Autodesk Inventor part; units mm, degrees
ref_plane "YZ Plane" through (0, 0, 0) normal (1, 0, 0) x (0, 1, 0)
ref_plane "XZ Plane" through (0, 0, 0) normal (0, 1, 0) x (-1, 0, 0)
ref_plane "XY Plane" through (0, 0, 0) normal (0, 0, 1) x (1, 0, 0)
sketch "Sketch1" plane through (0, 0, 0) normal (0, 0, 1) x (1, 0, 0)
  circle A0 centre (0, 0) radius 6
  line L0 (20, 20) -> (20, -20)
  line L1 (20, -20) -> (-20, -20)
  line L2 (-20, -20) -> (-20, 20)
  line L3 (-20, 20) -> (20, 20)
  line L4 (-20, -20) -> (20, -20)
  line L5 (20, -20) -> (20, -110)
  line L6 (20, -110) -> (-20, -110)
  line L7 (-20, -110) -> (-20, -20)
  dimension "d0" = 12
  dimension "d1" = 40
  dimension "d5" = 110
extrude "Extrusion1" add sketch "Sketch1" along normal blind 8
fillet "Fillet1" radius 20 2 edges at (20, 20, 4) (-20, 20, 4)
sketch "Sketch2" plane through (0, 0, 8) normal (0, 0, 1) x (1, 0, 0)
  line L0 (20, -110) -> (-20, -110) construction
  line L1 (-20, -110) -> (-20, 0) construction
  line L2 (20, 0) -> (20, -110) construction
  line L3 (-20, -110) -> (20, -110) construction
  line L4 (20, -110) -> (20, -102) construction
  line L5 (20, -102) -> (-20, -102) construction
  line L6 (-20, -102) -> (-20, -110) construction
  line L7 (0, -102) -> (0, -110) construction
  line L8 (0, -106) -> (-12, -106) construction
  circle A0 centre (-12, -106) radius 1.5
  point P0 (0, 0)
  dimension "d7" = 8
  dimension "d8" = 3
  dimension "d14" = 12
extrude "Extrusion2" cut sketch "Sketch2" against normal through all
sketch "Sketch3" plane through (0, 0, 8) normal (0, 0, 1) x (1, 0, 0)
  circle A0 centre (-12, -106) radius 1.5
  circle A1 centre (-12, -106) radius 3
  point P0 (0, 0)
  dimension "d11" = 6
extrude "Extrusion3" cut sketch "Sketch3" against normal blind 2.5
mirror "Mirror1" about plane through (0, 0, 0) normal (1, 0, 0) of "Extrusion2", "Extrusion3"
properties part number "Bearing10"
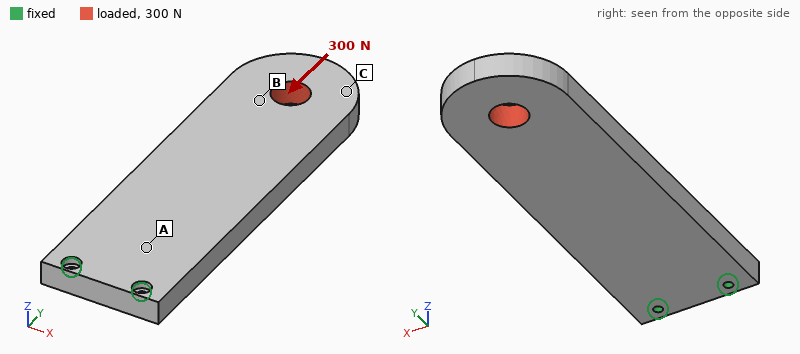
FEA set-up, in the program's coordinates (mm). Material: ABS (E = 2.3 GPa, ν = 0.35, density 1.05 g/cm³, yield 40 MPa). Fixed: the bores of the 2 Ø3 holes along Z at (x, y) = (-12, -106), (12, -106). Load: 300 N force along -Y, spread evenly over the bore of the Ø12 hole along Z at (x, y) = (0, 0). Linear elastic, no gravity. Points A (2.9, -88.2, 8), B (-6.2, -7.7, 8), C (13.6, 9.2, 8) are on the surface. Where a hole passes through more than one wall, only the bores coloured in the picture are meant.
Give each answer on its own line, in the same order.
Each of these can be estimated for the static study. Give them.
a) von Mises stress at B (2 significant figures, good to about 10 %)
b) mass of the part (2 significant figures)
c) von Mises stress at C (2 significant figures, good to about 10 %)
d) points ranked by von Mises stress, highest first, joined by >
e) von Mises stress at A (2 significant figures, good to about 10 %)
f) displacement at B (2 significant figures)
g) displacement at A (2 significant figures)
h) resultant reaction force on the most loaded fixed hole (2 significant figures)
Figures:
1.5 MPa
41 g
0.46 MPa
B > A > C
0.88 MPa
0.14 mm
0.030 mm
150 N
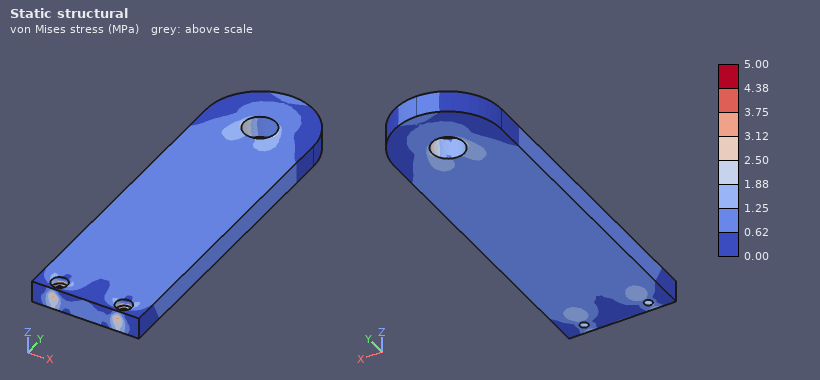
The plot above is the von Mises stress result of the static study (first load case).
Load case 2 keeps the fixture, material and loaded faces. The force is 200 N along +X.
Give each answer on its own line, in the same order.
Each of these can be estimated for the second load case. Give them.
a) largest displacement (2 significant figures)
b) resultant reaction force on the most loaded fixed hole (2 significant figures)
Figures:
1.5 mm
840 N
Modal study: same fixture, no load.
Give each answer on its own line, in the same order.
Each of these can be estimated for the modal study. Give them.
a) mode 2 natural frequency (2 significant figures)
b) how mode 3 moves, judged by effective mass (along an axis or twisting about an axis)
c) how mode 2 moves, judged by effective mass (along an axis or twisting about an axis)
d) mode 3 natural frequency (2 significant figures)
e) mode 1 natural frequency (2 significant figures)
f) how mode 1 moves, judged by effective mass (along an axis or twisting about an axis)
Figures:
530 Hz
along Z
along X
710 Hz
110 Hz
along Z
